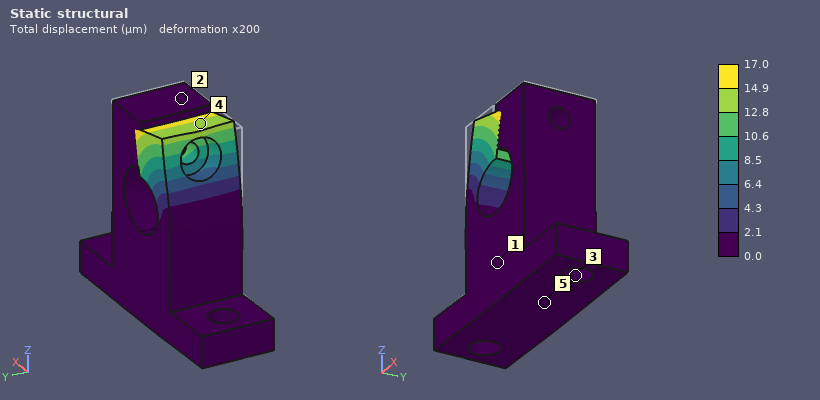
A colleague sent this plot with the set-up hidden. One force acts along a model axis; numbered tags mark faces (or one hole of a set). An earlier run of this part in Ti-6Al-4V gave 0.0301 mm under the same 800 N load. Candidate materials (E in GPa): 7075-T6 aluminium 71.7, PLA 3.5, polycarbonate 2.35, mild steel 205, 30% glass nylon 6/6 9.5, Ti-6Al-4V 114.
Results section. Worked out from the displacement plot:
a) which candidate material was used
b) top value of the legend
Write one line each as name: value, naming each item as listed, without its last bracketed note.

which candidate material was used: mild steel
top value of the legend: 17.0 µm
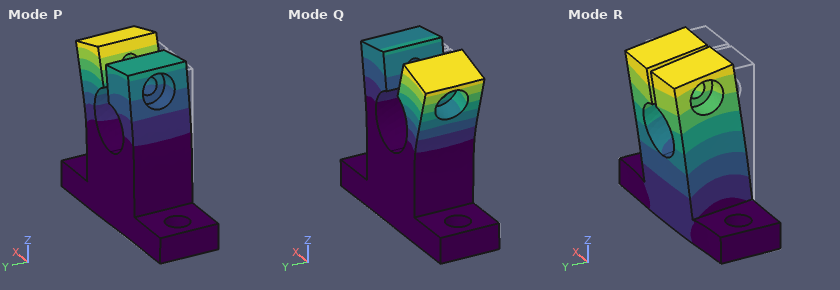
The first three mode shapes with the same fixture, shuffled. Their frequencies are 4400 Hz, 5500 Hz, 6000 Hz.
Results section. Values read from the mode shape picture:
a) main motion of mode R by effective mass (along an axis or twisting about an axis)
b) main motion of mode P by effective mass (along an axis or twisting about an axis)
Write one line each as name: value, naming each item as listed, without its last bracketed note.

main motion of mode R by effective mass: along Y
main motion of mode P by effective mass: along X
